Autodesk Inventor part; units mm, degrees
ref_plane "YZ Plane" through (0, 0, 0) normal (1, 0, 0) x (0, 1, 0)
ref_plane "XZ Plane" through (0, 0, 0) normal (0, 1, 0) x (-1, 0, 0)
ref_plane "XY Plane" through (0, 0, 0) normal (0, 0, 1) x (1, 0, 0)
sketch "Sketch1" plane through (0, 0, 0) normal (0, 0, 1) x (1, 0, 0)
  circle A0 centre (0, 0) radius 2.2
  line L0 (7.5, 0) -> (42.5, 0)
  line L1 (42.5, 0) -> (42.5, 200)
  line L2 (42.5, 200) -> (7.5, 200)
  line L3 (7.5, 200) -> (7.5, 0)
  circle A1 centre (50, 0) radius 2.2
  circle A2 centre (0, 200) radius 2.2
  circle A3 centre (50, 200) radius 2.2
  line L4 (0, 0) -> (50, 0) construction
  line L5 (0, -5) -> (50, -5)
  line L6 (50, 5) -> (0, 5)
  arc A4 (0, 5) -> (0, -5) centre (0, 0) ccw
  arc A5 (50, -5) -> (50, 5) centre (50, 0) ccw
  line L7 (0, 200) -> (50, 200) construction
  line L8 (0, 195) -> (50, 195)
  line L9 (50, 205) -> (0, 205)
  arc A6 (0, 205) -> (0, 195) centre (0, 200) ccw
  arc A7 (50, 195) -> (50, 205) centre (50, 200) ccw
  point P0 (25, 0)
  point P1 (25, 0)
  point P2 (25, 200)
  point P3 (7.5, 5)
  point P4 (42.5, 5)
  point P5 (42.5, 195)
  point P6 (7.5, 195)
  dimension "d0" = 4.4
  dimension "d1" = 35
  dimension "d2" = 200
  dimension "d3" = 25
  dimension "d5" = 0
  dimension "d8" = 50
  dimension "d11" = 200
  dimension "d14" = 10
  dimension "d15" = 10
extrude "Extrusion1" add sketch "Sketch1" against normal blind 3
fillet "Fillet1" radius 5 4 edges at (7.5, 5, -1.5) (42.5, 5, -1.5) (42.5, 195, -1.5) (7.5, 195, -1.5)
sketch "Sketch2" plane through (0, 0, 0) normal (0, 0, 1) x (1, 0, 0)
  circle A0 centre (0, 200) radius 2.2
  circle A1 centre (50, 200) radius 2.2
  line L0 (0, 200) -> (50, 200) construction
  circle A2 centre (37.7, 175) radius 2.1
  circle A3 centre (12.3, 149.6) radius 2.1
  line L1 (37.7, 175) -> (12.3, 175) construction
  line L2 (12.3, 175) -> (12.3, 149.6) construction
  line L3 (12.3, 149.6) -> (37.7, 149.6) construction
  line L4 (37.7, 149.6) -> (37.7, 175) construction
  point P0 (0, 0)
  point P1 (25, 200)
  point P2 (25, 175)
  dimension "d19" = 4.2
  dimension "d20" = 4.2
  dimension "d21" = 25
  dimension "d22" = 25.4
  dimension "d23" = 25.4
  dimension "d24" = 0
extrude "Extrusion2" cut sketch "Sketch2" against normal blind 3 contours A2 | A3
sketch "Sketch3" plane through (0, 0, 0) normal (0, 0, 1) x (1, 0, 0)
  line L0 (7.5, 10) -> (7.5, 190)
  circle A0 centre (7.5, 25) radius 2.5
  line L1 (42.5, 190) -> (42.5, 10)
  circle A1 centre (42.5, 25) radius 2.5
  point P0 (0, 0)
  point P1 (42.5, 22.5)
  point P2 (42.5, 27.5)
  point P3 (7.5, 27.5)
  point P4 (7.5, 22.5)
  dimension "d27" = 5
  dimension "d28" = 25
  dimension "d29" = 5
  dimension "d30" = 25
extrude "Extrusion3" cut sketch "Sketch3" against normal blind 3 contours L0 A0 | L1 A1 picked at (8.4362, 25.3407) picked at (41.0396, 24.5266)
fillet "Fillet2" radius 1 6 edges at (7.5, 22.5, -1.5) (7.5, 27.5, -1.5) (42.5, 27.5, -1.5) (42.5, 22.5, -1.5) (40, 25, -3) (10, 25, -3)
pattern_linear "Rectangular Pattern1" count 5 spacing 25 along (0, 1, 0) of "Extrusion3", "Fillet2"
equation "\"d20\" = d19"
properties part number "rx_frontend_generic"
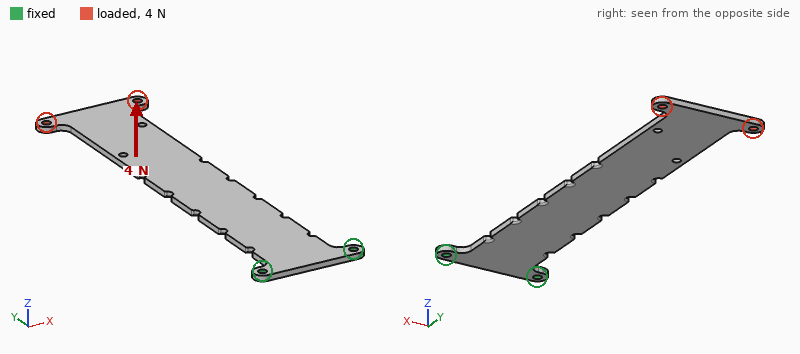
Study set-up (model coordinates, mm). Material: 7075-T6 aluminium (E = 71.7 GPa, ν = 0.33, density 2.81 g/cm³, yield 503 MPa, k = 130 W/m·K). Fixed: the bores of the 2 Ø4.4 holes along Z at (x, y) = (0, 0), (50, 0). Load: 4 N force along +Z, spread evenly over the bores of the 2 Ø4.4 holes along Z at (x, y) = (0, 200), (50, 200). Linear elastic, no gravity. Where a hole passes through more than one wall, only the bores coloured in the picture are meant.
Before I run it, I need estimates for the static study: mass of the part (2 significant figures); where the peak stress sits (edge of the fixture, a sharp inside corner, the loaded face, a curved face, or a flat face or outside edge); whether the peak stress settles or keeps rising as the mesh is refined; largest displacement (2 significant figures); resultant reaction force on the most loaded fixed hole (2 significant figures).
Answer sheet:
64 g
edge of the fixture
keeps rising
2.3 mm
2.0 N
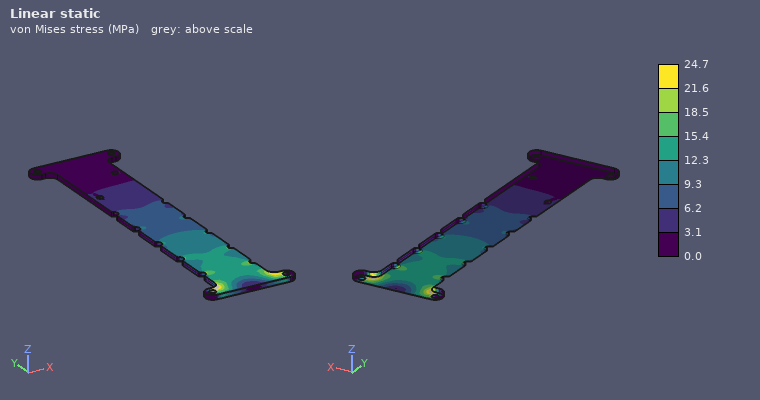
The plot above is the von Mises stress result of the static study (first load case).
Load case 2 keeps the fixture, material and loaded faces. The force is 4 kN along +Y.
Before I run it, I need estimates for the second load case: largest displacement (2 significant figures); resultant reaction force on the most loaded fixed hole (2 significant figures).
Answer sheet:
0.28 mm
2.3 kN
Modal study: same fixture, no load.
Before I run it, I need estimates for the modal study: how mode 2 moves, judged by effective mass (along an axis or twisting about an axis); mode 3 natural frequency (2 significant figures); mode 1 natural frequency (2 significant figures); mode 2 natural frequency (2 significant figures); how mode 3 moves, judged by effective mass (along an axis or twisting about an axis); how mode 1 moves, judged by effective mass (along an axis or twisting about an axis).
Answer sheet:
along Z
550 Hz
50 Hz
320 Hz
along X
along Z
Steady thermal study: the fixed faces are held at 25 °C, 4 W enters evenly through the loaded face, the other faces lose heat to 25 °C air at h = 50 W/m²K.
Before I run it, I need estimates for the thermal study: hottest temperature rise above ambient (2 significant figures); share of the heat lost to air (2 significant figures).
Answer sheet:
20 K
96 %
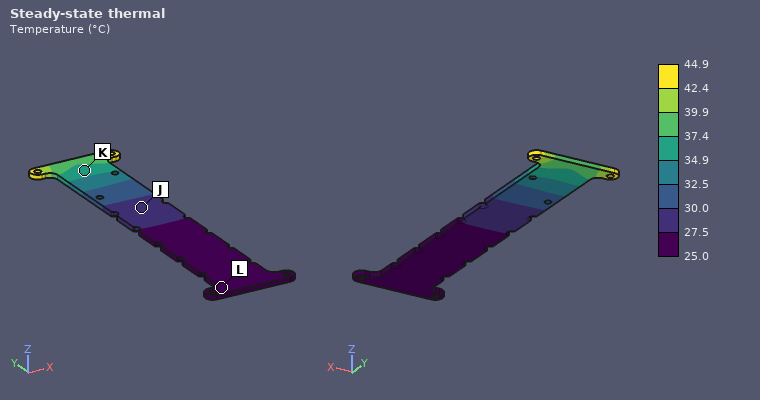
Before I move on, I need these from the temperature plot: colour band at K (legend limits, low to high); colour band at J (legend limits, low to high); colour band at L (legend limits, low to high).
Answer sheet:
34.9 to 37.4 °C
27.5 to 30.0 °C
25.0 to 27.5 °C
